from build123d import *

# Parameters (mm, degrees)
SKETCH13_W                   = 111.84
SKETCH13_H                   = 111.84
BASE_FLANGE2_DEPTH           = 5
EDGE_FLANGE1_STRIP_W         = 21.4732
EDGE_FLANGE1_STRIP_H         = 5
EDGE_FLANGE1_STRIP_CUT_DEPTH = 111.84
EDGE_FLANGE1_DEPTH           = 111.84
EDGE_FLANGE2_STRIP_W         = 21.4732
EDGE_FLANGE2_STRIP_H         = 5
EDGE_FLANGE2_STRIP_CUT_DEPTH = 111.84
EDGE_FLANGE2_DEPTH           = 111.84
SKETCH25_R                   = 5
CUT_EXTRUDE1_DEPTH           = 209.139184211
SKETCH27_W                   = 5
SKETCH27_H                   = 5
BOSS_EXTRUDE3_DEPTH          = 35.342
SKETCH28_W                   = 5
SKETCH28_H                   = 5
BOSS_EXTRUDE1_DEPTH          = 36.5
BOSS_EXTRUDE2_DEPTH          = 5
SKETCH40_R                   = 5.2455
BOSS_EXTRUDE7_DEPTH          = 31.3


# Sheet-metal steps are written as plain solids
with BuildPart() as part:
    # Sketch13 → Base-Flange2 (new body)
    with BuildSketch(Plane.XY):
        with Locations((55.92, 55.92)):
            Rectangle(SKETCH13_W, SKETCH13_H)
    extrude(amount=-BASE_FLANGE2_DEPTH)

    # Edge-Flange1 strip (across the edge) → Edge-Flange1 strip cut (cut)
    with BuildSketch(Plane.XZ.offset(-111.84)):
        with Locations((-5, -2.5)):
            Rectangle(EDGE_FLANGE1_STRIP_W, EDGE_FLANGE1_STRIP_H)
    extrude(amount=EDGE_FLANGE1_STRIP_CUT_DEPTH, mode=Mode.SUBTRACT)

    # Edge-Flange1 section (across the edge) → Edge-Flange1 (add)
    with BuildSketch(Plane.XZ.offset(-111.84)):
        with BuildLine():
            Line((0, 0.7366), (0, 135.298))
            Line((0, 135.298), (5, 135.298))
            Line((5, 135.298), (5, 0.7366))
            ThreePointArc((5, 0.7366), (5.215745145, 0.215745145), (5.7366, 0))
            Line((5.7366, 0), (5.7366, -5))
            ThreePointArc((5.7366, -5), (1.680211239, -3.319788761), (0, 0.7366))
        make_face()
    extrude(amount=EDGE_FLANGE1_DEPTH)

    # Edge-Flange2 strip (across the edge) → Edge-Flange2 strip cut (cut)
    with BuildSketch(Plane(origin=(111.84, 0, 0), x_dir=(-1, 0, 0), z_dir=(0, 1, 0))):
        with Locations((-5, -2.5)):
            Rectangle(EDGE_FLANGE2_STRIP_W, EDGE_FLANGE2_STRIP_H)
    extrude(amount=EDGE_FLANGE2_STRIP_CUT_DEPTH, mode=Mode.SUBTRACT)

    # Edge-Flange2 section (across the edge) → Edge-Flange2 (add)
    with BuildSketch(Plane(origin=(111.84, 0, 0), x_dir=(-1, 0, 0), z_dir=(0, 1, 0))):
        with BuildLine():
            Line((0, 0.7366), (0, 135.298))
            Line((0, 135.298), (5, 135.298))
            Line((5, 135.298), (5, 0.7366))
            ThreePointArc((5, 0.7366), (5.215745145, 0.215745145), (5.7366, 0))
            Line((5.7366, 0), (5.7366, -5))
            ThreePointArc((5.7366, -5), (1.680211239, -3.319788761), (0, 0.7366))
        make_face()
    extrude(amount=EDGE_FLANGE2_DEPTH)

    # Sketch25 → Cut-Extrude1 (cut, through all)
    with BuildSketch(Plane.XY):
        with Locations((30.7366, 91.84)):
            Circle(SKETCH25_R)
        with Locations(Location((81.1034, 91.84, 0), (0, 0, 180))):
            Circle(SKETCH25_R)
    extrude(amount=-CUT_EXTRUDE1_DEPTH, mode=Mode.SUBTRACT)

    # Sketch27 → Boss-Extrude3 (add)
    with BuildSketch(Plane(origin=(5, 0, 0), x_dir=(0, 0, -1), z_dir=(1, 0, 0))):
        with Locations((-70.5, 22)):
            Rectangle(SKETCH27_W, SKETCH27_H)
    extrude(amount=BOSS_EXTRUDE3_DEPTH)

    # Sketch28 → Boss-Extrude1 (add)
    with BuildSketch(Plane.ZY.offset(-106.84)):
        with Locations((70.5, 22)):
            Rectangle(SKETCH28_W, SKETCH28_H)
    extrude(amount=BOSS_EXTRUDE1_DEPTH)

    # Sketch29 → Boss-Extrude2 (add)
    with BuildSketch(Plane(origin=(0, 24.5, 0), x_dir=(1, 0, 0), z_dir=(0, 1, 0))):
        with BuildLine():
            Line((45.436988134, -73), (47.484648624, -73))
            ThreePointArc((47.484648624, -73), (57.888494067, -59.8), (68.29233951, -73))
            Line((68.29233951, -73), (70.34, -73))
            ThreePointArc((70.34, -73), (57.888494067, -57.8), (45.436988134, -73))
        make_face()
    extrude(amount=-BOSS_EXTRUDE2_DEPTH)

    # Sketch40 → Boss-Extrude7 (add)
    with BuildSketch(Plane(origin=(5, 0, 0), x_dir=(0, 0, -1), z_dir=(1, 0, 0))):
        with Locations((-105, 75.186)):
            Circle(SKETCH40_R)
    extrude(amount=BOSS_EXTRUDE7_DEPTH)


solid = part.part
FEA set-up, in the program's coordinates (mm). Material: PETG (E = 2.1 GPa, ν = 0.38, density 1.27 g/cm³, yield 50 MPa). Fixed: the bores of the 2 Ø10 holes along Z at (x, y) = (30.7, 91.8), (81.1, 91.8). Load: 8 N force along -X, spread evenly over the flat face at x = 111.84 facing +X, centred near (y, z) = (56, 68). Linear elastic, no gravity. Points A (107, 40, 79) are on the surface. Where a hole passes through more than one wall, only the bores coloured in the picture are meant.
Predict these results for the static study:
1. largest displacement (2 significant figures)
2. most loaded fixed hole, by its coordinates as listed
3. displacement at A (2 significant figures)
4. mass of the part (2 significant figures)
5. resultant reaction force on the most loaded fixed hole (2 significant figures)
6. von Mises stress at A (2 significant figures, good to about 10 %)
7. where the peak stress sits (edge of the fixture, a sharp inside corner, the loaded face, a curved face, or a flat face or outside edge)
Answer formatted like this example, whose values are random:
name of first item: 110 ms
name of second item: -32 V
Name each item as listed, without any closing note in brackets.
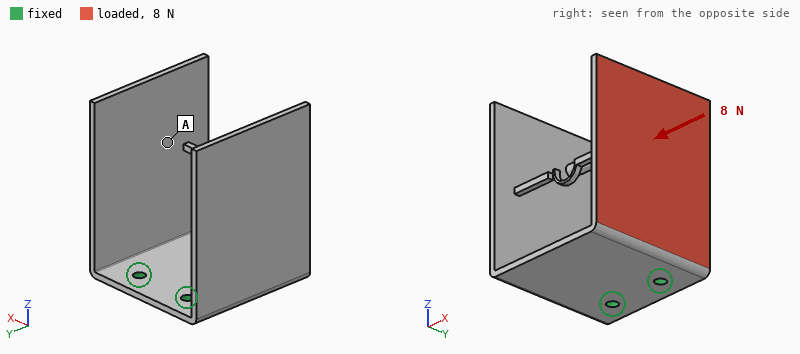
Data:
largest displacement: 2.1 mm
most loaded fixed hole, by its coordinates as listed: (81.1, 91.8)
displacement at A: 1.1 mm
mass of the part: 270 g
resultant reaction force on the most loaded fixed hole: 8.5 N
von Mises stress at A: 0.19 MPa
where the peak stress sits: a flat face or outside edge
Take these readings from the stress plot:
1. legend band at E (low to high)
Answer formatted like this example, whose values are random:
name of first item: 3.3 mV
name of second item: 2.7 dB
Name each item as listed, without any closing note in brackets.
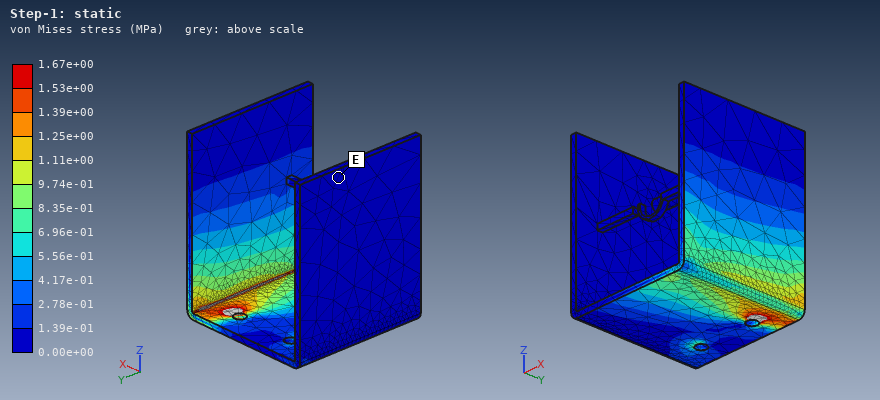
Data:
legend band at E: 0.00e+00 to 1.39e-01 MPa
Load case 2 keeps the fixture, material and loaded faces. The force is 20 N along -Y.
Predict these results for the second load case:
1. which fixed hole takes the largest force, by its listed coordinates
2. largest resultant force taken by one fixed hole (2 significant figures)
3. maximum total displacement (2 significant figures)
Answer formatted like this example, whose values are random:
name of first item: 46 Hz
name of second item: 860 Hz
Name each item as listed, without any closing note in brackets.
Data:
which fixed hole takes the largest force, by its listed coordinates: (81.1, 91.8)
largest resultant force taken by one fixed hole: 29 N
maximum total displacement: 2.1 mm
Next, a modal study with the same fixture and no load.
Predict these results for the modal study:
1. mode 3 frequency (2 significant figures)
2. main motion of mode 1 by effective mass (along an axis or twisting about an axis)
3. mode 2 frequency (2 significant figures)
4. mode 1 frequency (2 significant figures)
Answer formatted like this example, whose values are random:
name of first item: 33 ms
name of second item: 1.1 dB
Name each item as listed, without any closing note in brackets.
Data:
mode 3 frequency: 54 Hz
main motion of mode 1 by effective mass: along X
mode 2 frequency: 39 Hz
mode 1 frequency: 37 Hz
